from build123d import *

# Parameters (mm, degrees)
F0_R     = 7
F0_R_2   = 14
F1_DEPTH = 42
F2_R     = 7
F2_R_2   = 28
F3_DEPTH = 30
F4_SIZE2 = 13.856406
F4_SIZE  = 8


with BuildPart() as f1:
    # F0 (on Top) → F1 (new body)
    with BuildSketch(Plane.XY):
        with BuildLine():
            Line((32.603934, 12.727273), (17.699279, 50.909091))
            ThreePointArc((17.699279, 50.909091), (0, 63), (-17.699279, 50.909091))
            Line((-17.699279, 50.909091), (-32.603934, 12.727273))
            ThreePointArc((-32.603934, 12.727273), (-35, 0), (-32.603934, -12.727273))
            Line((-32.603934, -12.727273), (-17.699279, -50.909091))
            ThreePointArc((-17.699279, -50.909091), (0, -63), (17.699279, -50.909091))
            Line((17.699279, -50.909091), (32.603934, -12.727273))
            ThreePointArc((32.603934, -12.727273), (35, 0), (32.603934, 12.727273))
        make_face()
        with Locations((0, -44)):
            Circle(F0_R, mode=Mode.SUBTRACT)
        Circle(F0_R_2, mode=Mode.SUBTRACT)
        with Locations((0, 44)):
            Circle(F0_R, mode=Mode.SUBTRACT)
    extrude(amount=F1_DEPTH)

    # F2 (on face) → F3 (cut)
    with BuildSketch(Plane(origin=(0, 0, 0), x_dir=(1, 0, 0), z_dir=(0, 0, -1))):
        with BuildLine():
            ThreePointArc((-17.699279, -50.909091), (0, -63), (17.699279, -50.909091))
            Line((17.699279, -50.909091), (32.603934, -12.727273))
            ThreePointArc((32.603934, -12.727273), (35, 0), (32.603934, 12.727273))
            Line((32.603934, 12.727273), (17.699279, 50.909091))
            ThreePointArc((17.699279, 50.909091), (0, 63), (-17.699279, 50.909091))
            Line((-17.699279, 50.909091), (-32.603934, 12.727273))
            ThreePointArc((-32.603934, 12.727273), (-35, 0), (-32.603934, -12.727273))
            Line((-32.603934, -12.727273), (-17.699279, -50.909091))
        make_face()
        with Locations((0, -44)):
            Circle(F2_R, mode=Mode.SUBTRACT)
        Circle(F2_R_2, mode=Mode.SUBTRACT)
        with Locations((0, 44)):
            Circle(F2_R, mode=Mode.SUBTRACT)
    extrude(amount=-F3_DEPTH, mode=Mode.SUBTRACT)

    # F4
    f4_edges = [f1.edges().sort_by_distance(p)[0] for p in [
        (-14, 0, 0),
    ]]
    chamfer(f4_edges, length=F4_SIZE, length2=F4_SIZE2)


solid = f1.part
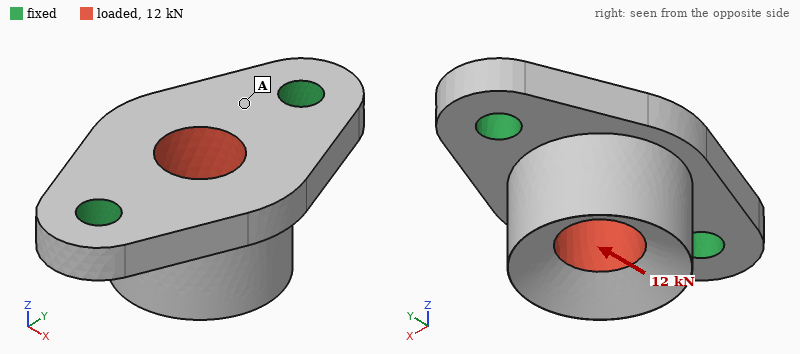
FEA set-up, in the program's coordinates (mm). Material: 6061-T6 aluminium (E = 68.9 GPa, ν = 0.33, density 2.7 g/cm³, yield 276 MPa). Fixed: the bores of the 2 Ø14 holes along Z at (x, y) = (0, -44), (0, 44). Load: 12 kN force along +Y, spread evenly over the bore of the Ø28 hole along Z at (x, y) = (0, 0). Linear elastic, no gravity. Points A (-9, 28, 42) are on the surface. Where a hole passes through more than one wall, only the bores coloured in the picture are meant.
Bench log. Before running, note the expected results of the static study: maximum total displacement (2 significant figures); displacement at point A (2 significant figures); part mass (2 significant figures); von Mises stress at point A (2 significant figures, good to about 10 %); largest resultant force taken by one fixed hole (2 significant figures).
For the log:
14 µm
4.3 µm
300 g
6.2 MPa
6.3 kN
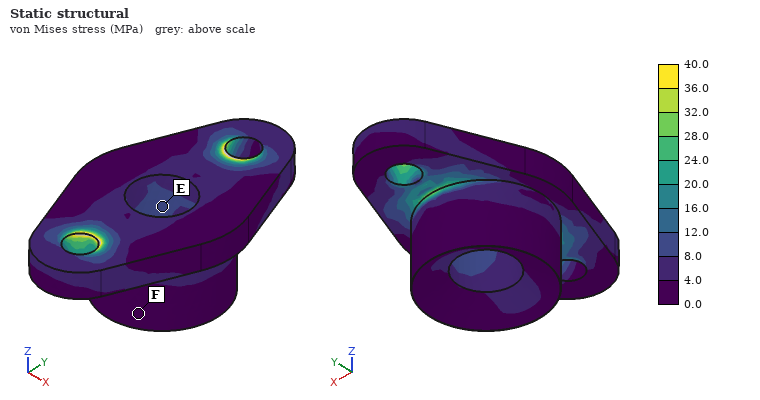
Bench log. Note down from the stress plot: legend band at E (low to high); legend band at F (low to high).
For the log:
8.0 to 12.0 MPa
0.0 to 4.0 MPa
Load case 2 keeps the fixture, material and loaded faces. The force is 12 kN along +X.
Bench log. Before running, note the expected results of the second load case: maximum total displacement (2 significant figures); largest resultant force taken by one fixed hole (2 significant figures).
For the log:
86 µm
6.0 kN
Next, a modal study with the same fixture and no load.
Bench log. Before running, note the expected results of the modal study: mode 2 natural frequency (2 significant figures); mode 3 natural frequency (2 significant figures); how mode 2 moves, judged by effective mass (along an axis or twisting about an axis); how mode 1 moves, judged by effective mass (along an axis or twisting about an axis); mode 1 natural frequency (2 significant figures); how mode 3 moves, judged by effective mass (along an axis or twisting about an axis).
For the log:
7000 Hz
11 kHz
along Z
along X
3900 Hz
along Y
